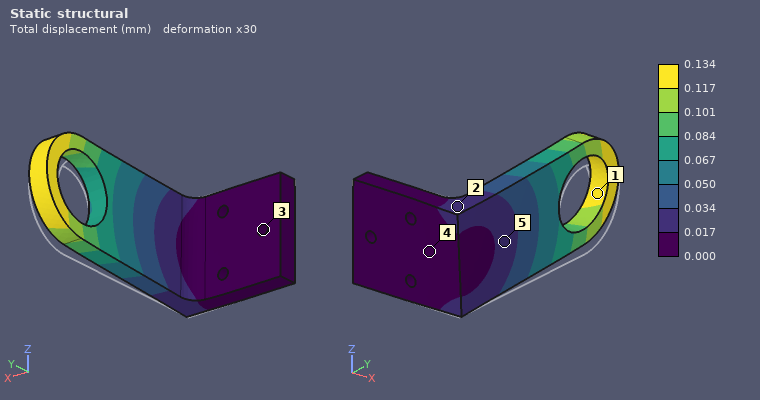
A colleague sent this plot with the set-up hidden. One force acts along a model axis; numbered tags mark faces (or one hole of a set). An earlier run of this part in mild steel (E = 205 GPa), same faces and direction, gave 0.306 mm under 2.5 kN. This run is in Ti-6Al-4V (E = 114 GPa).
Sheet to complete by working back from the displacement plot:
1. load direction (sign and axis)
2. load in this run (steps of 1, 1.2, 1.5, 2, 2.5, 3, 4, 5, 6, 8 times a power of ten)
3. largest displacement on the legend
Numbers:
+Z
600 N
0.134 mm
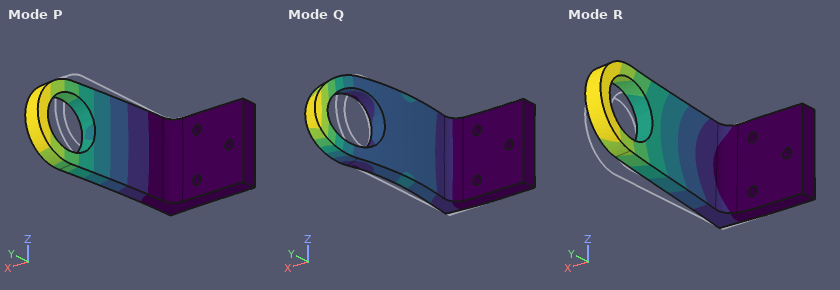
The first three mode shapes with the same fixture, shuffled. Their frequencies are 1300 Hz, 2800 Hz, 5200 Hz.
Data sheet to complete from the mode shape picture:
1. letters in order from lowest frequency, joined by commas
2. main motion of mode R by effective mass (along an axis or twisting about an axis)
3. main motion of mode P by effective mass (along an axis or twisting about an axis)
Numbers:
P, R, Q
along Z
along X
